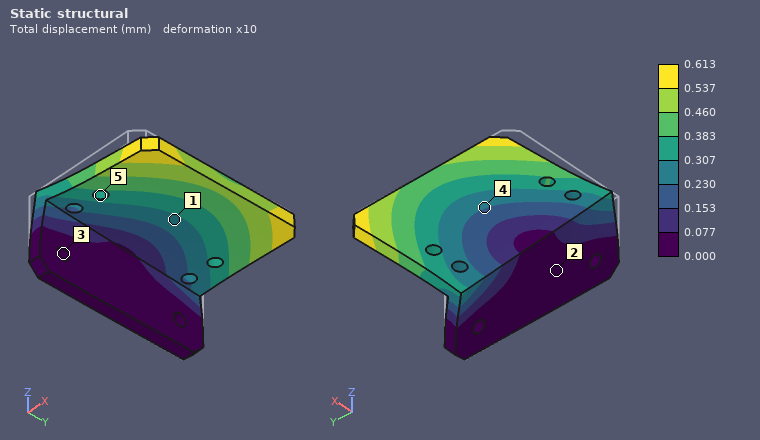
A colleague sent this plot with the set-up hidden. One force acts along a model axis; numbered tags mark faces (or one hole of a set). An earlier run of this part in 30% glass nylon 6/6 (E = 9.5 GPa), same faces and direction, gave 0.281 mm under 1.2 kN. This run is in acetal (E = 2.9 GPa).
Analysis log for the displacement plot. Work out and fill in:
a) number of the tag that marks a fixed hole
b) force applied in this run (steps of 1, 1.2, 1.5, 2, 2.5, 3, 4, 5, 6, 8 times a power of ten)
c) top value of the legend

3
800 N
0.613 mm
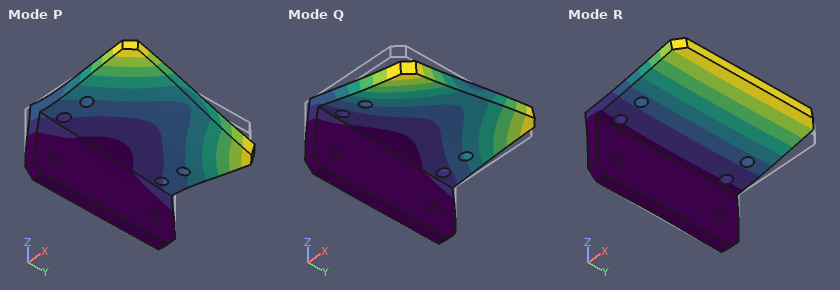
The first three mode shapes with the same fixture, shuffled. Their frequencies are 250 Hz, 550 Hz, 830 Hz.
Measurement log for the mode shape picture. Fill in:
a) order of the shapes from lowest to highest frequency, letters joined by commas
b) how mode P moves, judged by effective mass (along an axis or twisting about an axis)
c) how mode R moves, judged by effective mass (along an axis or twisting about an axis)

R, Q, P
along Y
along Z
